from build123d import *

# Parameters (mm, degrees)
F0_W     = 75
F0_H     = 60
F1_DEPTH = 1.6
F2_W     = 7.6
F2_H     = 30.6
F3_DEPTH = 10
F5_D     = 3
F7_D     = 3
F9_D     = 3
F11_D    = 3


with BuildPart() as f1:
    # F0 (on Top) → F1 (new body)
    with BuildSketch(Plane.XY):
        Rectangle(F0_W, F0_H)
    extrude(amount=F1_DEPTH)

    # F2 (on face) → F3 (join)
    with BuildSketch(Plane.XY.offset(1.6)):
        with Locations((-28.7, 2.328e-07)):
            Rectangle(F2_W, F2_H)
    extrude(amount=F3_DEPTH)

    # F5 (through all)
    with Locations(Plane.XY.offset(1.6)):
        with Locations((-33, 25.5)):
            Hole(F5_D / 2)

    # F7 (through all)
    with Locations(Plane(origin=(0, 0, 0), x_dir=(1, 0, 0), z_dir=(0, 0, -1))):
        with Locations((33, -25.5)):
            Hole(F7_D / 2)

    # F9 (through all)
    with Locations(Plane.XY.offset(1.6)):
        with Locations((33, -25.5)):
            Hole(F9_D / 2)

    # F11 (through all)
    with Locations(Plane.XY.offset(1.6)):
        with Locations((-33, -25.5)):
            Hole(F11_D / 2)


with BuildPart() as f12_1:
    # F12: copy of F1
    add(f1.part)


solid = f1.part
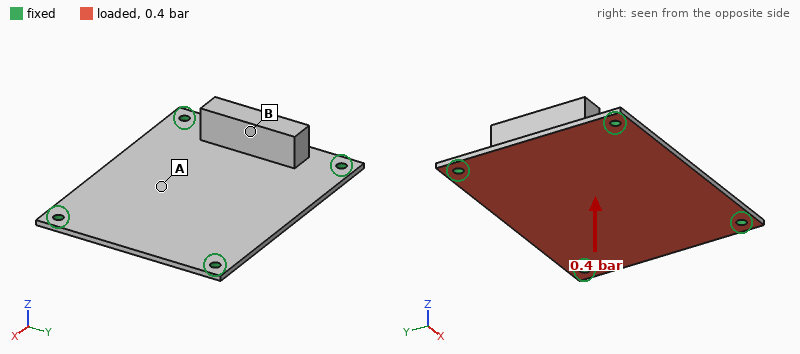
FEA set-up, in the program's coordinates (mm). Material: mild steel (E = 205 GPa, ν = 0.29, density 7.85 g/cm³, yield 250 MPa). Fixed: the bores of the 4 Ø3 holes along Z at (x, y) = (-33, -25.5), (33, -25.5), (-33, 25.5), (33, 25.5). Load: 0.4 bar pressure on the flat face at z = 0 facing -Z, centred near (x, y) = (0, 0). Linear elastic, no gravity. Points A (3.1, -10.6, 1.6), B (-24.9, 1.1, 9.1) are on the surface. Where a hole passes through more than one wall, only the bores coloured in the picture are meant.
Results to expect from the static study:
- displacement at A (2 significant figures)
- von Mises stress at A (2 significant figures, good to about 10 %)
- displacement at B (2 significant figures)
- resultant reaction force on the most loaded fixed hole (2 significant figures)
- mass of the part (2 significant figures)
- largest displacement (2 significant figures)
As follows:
43 µm
18 MPa
18 µm
47 N
74 g
45 µm
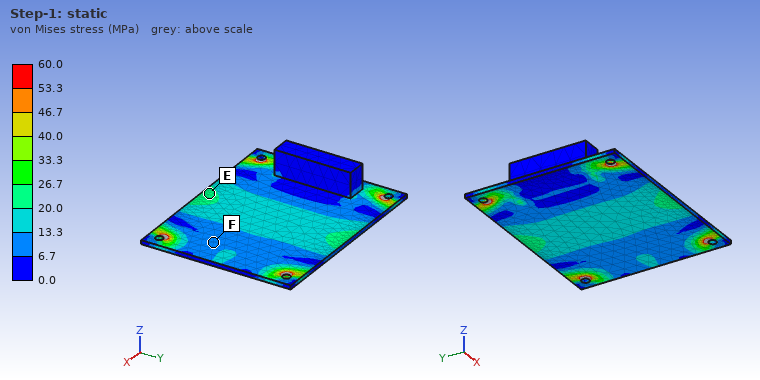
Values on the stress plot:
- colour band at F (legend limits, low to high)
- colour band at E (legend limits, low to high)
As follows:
6.7 to 13.3 MPa
20.0 to 26.7 MPa
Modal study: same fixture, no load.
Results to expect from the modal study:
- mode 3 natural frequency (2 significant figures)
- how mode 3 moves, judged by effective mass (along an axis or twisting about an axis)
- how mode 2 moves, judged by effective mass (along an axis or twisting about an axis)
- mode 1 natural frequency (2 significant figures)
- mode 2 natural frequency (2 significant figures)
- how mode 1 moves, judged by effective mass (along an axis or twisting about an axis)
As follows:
3200 Hz
twisting about Y
twisting about X
1500 Hz
2600 Hz
along Z
